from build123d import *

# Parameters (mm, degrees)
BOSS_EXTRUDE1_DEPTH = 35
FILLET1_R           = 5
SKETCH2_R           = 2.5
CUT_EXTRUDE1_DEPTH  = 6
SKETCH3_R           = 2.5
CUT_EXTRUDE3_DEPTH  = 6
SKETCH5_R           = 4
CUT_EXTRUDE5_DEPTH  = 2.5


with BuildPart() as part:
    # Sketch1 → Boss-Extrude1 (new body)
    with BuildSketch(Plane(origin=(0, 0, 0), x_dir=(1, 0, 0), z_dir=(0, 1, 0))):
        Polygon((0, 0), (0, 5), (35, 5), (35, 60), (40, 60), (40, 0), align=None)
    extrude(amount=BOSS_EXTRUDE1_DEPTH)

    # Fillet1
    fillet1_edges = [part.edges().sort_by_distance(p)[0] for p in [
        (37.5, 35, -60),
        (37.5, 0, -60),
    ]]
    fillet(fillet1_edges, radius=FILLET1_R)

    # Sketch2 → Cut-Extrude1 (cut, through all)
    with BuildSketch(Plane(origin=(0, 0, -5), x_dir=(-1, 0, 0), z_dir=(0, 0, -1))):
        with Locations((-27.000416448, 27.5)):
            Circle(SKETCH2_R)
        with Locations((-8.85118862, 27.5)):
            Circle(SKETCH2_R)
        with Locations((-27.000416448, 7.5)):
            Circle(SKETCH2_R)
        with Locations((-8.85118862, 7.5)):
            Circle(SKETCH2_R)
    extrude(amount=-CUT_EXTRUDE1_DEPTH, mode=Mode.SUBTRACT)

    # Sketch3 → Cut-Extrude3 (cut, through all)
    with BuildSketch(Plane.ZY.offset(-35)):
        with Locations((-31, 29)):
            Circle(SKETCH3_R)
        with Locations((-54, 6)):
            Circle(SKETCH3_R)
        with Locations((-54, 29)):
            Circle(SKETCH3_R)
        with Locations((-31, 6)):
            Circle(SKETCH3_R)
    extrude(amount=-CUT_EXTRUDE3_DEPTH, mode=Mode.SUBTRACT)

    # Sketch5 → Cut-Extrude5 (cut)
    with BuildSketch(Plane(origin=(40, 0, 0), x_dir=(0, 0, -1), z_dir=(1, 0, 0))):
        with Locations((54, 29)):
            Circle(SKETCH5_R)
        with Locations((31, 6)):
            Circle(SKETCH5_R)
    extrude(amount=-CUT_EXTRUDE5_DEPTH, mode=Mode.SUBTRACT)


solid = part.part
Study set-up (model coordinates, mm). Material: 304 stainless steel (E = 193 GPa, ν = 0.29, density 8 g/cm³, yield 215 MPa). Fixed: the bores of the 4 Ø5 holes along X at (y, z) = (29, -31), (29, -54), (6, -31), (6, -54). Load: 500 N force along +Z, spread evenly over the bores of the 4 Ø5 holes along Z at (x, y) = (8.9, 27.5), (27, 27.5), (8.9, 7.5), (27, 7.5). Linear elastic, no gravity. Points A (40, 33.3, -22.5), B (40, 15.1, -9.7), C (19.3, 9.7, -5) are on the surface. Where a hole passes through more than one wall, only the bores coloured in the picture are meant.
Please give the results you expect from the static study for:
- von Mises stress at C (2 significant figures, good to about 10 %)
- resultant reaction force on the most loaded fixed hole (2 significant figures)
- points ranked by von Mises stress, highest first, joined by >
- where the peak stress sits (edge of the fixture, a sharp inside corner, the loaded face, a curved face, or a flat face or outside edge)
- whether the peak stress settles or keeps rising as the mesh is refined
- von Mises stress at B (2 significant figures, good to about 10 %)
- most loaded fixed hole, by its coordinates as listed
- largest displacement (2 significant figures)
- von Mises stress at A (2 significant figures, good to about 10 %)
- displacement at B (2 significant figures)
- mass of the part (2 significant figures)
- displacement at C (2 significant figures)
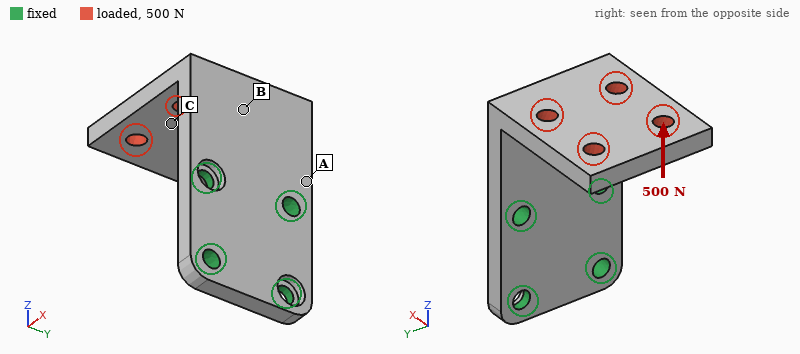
17 MPa
460 N
A > B > C
edge of the fixture
keeps rising
56 MPa
(6, -31)
0.20 mm
72 MPa
0.035 mm
130 g
0.097 mm
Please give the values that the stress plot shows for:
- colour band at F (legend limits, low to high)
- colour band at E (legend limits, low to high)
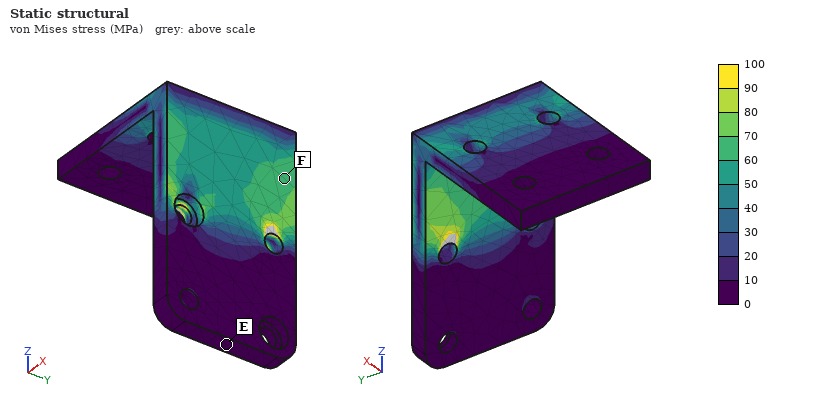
60 to 70 MPa
0 to 10 MPa
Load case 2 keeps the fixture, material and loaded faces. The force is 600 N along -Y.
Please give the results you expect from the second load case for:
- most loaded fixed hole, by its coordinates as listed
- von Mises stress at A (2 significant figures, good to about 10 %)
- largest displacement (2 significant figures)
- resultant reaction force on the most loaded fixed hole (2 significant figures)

(29, -31)
50 MPa
94 µm
800 N
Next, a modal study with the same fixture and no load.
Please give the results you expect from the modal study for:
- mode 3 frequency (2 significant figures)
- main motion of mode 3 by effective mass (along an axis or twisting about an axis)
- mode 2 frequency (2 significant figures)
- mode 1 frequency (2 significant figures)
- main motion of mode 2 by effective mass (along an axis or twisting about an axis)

3400 Hz
along X
2200 Hz
1200 Hz
along Y
